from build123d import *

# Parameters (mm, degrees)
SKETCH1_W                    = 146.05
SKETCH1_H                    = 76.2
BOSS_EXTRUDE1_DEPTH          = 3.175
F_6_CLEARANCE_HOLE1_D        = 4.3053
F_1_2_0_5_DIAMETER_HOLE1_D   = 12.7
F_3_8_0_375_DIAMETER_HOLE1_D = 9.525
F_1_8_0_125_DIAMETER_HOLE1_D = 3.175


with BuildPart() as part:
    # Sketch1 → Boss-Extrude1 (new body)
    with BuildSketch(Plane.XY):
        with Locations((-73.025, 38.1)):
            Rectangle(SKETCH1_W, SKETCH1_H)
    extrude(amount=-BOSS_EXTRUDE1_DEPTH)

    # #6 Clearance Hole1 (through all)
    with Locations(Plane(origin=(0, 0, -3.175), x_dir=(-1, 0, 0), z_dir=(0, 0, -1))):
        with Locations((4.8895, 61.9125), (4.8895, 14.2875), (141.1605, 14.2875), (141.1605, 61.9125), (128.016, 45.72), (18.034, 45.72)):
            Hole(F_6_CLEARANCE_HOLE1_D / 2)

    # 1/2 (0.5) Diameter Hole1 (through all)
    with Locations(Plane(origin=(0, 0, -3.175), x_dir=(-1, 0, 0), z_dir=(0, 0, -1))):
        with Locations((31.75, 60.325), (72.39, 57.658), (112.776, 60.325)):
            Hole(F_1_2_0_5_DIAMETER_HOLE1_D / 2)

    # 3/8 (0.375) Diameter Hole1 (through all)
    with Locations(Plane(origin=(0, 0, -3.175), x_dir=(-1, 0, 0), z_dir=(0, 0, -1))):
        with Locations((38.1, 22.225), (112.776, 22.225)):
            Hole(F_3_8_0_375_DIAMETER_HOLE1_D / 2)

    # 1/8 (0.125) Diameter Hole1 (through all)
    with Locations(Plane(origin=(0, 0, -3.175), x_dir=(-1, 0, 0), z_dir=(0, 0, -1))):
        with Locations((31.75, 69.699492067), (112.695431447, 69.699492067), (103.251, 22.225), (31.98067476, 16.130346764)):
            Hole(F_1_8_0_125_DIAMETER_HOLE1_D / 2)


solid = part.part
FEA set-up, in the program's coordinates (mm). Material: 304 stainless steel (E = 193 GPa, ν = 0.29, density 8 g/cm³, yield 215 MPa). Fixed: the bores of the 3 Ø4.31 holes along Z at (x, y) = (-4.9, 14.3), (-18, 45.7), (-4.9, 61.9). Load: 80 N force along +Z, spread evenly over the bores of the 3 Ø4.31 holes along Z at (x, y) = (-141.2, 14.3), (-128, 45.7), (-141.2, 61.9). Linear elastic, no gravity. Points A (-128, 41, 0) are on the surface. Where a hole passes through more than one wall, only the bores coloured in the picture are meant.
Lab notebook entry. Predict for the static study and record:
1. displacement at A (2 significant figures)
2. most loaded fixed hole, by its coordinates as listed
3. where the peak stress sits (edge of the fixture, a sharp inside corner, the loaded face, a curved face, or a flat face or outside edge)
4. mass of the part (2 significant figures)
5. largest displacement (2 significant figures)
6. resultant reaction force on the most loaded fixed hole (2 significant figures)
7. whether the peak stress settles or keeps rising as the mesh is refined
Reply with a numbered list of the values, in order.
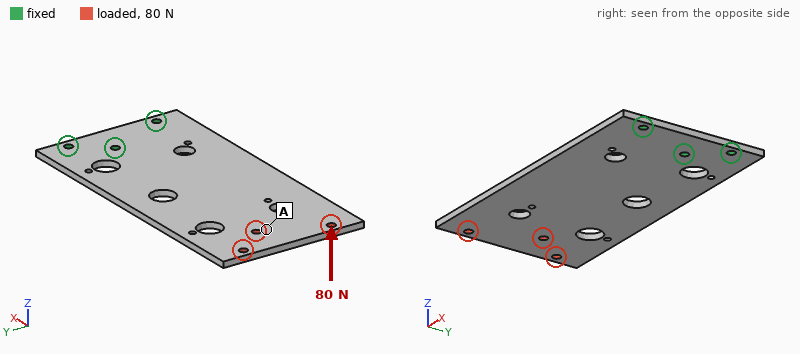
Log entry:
1. 1.3 mm
2. (-18, 45.7)
3. edge of the fixture
4. 270 g
5. 1.6 mm
6. 300 N
7. keeps rising
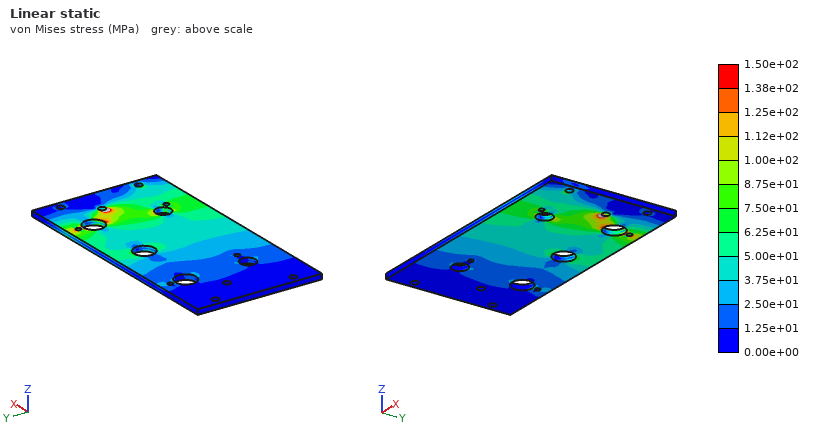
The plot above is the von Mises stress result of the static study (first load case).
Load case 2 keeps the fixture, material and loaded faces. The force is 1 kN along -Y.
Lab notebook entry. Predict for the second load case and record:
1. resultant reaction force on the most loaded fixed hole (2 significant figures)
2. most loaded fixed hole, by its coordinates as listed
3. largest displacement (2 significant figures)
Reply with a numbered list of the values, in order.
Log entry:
1. 2.4 kN
2. (-4.9, 14.3)
3. 67 µm
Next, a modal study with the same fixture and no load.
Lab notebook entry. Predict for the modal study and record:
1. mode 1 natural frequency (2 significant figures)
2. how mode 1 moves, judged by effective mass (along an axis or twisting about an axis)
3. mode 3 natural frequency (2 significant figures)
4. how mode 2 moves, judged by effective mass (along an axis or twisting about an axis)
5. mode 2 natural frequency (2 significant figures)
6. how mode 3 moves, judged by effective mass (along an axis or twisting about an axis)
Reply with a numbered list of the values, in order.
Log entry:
1. 140 Hz
2. along Z
3. 860 Hz
4. twisting about X
5. 510 Hz
6. along Z
